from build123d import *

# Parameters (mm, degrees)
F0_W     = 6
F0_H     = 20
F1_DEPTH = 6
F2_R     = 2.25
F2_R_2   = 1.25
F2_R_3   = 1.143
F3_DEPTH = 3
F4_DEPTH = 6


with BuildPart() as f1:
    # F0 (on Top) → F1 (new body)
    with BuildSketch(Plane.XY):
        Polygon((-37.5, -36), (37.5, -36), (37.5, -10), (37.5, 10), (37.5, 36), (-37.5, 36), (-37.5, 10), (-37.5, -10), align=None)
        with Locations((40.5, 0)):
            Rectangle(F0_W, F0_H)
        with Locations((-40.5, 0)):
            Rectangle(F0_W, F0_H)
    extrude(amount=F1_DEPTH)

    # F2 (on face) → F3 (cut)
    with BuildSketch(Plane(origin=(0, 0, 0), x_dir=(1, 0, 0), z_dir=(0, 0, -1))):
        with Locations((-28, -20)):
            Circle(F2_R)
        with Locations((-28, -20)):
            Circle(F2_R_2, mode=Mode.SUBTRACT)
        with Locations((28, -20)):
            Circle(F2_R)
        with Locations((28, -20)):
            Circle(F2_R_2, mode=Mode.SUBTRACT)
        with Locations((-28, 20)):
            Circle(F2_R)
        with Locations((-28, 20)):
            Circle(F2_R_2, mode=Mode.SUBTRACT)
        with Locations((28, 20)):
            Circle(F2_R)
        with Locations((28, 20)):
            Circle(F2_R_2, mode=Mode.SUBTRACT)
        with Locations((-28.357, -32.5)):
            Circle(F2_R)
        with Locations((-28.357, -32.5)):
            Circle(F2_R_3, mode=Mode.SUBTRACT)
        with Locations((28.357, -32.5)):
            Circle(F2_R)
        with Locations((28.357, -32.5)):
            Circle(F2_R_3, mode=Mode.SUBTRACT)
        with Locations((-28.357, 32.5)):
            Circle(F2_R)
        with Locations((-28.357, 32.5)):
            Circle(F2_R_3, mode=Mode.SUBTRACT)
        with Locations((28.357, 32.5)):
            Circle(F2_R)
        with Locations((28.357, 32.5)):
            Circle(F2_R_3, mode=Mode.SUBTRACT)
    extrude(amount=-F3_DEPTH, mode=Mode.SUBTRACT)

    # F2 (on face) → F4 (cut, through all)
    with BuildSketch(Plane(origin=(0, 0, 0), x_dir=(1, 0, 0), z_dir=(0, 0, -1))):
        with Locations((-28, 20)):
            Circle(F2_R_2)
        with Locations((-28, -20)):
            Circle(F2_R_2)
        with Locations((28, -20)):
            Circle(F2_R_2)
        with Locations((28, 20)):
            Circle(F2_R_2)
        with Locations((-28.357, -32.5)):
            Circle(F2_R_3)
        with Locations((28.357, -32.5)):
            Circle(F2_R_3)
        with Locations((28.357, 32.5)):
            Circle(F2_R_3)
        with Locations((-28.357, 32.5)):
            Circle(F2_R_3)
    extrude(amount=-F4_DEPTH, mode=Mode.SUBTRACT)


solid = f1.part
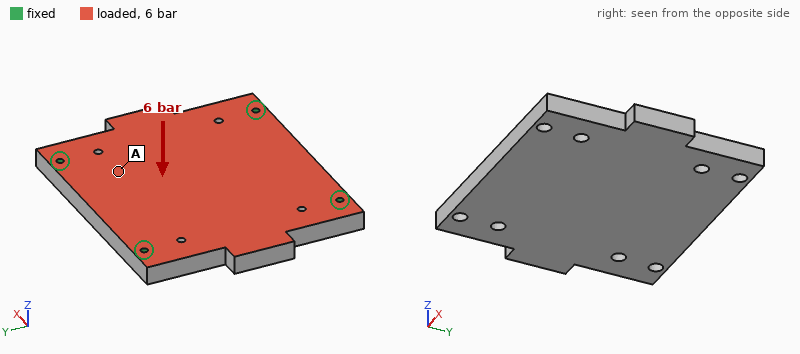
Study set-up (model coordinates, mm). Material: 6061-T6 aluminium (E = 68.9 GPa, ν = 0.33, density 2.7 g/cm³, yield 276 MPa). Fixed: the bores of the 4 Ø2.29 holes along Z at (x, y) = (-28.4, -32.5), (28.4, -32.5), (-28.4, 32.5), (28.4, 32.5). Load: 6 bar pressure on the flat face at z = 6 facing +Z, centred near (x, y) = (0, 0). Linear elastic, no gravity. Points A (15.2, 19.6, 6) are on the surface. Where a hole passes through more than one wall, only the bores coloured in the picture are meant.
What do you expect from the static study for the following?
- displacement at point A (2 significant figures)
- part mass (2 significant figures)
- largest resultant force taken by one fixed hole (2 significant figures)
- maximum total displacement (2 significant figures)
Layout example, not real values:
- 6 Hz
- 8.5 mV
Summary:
- 56 µm
- 90 g
- 1.2 kN
- 86 µm
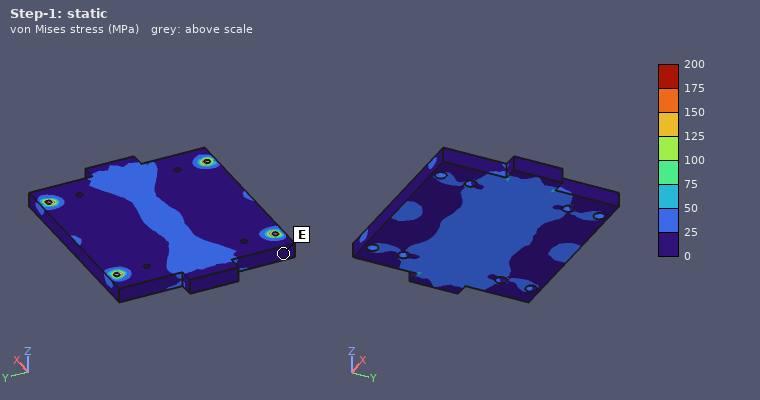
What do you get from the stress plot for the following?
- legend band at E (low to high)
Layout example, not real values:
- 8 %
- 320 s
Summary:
- 0 to 25 MPa
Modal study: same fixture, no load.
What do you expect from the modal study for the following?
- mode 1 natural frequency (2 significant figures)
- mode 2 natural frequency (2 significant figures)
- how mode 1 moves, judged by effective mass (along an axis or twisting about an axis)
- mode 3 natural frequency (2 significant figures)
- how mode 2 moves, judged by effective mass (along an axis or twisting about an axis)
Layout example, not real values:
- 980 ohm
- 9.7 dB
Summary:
- 3800 Hz
- 5100 Hz
- along Z
- 5900 Hz
- twisting about Y
